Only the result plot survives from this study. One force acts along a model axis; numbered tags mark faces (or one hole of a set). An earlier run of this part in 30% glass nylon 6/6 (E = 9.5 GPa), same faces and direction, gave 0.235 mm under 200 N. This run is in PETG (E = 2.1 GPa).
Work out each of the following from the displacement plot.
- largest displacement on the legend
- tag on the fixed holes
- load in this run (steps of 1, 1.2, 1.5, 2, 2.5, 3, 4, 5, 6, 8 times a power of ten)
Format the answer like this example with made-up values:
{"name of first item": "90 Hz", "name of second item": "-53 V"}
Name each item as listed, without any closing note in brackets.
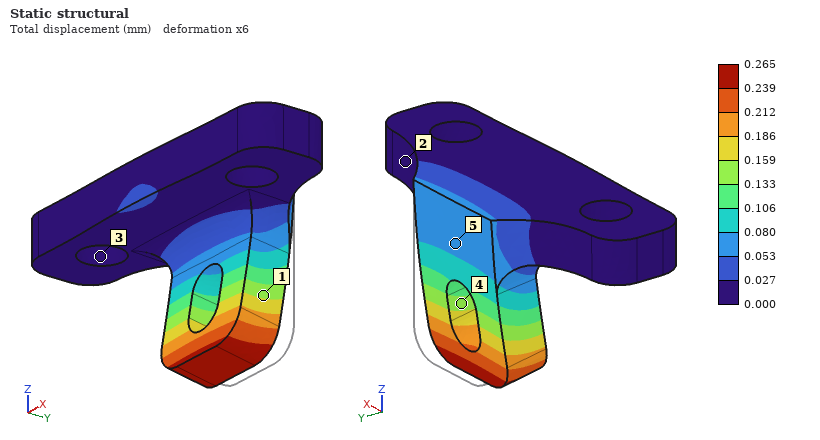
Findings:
{"largest displacement on the legend": "0.265 mm", "tag on the fixed holes": "3", "load in this run": "50 N"}
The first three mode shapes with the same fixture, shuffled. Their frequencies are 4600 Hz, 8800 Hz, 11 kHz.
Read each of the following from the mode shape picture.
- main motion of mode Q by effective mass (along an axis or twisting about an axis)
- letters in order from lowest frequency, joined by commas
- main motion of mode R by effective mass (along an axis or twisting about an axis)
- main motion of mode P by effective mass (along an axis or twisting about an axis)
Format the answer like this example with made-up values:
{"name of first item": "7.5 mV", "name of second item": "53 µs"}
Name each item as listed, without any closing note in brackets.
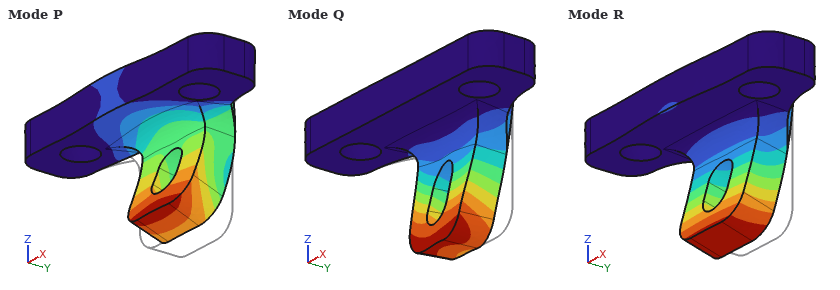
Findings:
{"main motion of mode Q by effective mass": "along X", "letters in order from lowest frequency, joined by commas": "R, Q, P", "main motion of mode R by effective mass": "along Y", "main motion of mode P by effective mass": "along Z"}
